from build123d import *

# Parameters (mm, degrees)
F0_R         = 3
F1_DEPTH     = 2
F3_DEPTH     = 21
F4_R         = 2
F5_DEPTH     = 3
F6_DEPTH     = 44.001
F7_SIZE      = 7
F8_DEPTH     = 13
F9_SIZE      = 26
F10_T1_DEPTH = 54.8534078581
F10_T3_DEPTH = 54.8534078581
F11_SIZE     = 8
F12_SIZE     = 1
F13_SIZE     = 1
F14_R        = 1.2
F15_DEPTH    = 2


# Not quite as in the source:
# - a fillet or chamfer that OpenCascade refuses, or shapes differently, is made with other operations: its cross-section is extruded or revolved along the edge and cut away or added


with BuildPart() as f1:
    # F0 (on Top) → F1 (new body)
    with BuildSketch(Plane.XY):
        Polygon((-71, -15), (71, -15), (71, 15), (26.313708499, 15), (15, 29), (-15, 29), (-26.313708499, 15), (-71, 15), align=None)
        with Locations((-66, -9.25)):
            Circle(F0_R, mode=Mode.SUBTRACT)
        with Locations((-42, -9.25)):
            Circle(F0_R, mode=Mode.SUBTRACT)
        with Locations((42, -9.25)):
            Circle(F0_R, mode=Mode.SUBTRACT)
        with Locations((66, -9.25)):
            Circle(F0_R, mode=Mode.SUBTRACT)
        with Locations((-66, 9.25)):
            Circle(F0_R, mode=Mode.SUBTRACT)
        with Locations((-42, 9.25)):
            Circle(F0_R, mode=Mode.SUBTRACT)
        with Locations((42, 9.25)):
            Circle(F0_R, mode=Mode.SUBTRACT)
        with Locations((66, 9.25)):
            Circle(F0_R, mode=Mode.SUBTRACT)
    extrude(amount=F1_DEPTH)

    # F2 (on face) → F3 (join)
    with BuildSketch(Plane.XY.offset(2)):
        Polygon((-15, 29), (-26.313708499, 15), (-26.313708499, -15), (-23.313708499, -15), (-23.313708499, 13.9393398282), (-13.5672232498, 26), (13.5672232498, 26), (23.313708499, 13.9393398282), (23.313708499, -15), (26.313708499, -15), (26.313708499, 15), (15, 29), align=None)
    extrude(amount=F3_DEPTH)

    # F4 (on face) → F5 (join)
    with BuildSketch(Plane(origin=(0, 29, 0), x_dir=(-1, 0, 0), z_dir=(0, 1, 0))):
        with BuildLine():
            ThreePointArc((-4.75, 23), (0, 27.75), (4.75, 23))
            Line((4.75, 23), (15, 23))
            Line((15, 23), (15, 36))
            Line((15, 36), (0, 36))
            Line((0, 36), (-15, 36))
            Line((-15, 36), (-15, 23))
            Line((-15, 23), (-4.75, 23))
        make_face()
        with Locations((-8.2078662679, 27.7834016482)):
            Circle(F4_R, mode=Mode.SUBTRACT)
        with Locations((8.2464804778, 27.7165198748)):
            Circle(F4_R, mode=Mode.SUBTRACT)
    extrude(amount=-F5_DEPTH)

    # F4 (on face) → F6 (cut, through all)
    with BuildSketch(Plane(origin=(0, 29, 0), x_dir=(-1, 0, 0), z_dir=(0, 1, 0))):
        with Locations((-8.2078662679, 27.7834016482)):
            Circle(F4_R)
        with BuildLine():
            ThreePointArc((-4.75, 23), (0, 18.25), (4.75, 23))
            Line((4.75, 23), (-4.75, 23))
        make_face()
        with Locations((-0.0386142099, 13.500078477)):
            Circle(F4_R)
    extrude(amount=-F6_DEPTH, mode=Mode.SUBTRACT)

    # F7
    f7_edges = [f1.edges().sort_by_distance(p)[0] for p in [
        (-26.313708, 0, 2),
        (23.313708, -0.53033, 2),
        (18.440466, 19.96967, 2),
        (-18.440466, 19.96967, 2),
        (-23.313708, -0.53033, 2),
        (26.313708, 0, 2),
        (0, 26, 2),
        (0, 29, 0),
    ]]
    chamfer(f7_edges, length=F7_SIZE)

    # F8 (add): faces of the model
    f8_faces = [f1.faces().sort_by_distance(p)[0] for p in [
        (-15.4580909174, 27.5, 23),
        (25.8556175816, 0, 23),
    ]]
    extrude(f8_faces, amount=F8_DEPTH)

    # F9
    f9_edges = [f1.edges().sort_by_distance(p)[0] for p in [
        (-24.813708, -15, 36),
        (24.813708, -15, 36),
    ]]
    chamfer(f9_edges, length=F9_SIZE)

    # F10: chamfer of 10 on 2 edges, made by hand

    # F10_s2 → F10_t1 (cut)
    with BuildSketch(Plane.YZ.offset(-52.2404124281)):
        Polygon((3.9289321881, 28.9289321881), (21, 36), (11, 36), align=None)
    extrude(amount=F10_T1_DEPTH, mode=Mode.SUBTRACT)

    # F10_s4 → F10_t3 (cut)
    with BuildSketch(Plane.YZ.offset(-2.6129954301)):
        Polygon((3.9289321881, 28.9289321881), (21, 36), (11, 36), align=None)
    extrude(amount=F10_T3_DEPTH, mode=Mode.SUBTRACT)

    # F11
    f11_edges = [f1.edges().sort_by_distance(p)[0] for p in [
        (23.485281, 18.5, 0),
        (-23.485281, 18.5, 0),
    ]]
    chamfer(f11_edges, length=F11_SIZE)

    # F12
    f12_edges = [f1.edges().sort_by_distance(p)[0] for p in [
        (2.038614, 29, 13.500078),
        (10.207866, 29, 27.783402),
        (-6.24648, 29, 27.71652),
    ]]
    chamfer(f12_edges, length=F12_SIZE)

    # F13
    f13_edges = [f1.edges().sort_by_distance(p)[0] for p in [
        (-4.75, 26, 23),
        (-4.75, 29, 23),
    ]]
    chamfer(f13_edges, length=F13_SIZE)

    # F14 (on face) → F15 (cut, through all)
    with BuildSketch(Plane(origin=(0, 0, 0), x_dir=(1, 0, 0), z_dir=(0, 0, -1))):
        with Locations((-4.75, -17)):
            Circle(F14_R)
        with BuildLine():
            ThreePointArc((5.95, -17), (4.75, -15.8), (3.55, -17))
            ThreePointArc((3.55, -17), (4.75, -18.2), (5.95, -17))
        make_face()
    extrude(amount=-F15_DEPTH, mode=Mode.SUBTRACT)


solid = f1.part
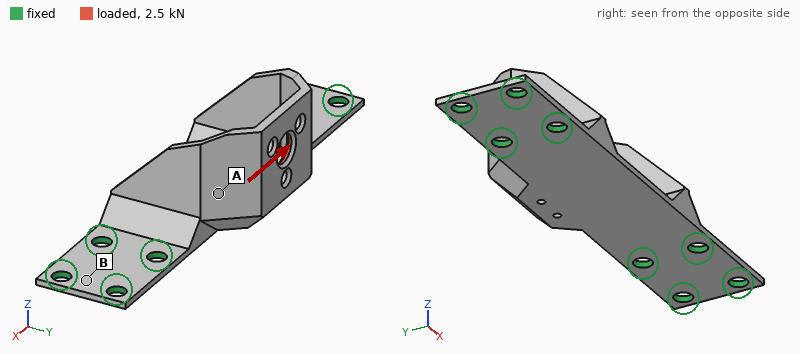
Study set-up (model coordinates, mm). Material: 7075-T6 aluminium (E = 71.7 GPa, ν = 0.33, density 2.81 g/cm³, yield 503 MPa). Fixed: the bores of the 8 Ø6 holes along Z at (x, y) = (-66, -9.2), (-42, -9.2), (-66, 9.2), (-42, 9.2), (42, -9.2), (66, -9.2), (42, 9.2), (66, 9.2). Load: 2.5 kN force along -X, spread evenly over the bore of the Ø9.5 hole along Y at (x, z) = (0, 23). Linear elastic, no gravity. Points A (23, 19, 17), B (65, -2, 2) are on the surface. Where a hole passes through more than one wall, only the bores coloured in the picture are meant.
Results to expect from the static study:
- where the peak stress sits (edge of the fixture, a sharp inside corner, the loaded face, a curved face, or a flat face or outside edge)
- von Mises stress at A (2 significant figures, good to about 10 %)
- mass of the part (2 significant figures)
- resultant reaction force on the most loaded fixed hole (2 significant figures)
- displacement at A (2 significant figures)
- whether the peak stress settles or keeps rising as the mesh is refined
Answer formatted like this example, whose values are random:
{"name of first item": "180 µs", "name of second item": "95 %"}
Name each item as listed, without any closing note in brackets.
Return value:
{"where the peak stress sits": "edge of the fixture", "von Mises stress at A": "49 MPa", "mass of the part": "60 g", "resultant reaction force on the most loaded fixed hole": "1.2 kN", "displacement at A": "0.13 mm", "whether the peak stress settles or keeps rising as the mesh is refined": "keeps rising"}
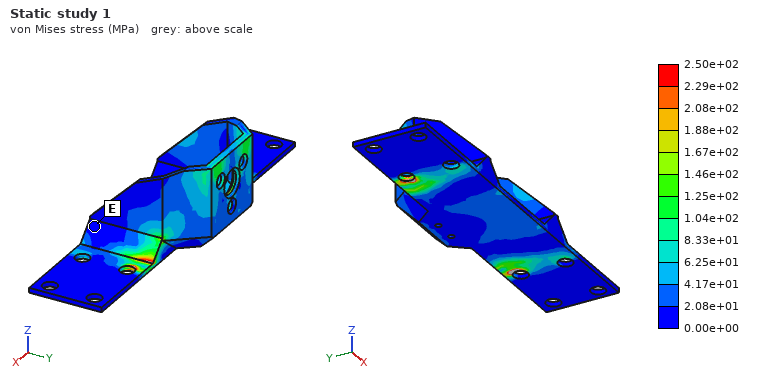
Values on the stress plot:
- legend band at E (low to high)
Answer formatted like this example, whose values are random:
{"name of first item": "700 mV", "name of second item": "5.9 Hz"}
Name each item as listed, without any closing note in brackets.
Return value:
{"legend band at E": "0.00e+00 to 2.08e+01 MPa"}
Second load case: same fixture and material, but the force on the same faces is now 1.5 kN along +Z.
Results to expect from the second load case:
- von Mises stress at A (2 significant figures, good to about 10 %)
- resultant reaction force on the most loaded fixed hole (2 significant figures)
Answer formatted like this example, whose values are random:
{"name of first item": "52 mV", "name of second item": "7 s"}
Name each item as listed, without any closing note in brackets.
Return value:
{"von Mises stress at A": "88 MPa", "resultant reaction force on the most loaded fixed hole": "1.8 kN"}
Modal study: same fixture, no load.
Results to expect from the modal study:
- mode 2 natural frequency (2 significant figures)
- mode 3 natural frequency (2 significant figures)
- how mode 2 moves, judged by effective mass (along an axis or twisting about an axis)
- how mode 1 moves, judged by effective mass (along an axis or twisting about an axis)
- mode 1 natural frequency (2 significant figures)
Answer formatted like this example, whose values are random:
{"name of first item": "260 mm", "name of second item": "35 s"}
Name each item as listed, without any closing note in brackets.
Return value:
{"mode 2 natural frequency": "2900 Hz", "mode 3 natural frequency": "3300 Hz", "how mode 2 moves, judged by effective mass": "along Z", "how mode 1 moves, judged by effective mass": "along Z", "mode 1 natural frequency": "1800 Hz"}
